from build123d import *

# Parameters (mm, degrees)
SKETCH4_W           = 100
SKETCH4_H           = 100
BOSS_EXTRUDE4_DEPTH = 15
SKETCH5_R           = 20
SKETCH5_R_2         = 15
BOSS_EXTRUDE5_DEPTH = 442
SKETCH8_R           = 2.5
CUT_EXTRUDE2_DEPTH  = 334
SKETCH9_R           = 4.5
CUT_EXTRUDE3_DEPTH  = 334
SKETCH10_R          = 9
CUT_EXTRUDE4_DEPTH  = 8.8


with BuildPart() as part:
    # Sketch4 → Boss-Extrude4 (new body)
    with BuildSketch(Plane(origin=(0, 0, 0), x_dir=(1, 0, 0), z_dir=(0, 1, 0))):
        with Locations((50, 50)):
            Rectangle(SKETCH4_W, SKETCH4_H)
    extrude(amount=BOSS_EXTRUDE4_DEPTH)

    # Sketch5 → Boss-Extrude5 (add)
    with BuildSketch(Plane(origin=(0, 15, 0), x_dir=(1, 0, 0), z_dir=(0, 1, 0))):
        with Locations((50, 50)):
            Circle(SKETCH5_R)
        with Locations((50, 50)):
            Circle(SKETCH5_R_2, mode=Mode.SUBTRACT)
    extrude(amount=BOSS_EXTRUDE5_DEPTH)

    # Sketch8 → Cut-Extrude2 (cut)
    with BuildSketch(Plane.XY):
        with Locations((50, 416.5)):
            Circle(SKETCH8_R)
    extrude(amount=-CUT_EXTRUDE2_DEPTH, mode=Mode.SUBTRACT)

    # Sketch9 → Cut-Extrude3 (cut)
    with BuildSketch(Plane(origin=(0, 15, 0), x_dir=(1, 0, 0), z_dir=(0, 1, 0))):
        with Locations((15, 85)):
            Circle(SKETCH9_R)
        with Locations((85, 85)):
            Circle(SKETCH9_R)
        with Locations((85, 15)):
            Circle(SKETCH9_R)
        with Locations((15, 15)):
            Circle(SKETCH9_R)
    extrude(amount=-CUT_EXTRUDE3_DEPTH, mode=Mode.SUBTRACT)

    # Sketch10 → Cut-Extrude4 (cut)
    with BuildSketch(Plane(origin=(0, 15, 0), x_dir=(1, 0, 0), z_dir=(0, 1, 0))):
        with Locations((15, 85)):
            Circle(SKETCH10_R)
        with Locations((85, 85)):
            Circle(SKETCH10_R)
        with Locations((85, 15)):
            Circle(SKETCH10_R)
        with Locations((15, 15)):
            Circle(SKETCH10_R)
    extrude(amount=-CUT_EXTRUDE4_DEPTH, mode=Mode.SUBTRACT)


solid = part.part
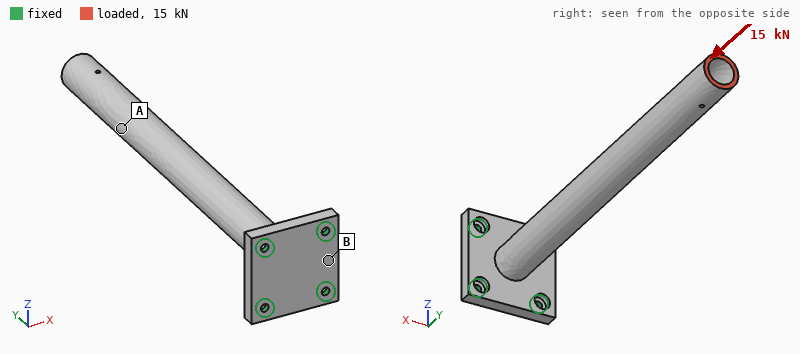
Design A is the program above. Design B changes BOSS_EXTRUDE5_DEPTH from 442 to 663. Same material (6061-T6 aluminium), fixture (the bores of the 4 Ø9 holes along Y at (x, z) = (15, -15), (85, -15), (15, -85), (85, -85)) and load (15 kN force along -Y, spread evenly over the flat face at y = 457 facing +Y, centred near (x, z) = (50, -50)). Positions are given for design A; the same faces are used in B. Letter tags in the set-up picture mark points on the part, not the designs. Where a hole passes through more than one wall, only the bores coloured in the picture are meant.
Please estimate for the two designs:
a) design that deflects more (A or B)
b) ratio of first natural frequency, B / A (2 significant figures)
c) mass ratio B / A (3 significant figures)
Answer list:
B
0.46
1.32
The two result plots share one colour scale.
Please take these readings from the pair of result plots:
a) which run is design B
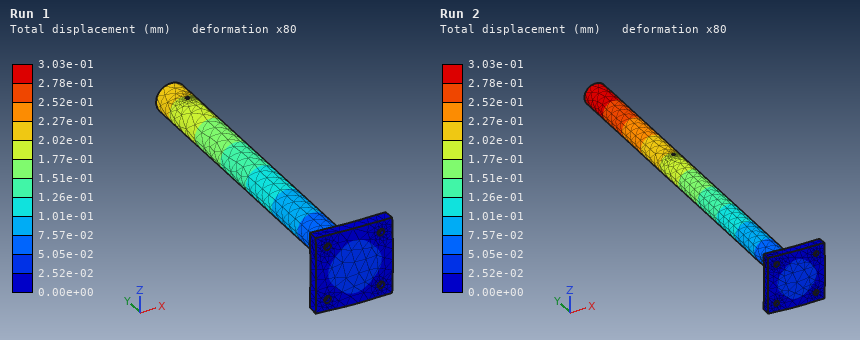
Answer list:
Run 2
